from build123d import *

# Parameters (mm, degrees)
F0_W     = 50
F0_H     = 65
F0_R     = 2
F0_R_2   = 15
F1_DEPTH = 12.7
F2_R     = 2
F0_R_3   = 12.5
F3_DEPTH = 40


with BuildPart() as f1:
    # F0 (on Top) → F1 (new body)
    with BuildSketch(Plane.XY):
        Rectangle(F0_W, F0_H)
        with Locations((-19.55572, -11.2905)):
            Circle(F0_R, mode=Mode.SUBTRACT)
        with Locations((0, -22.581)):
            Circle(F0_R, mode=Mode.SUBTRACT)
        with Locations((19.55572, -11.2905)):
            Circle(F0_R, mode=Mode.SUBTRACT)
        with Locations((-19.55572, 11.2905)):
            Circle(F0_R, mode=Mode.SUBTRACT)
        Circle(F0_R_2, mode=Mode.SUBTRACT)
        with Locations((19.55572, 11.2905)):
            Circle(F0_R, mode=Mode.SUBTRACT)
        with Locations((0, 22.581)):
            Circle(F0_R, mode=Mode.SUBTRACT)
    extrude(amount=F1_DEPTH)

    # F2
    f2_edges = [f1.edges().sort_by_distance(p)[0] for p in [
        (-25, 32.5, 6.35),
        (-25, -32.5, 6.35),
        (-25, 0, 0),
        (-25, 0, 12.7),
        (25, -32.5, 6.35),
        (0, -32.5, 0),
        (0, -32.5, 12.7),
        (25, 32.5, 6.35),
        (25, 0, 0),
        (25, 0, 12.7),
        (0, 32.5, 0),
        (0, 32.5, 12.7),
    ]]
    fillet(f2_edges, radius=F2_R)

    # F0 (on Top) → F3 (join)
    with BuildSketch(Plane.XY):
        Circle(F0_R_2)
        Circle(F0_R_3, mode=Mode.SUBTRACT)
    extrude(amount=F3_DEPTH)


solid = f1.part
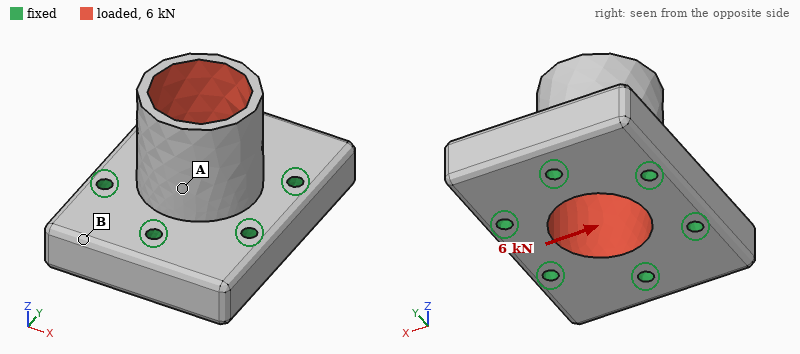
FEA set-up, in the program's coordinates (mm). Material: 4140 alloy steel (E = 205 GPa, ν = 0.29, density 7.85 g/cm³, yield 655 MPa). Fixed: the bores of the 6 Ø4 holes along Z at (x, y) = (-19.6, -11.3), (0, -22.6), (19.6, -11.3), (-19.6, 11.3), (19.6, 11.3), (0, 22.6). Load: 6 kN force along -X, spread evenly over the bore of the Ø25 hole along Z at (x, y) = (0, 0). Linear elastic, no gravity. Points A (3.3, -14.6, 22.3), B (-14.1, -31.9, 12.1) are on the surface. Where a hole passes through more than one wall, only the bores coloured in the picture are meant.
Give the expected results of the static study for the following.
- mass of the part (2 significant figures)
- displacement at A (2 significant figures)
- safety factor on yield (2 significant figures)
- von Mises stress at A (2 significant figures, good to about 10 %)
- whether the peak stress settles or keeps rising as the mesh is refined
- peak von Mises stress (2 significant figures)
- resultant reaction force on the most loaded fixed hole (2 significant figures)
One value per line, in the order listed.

310 g
5.6 µm
11
37 MPa
settles
60 MPa
1.6 kN
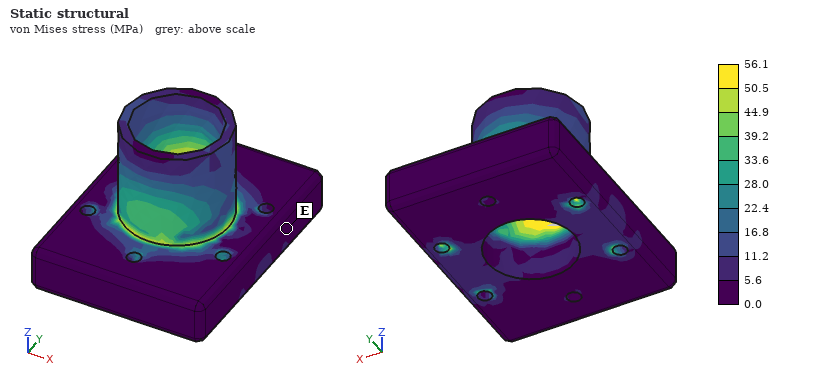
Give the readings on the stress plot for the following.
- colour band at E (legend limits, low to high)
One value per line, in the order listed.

0.0 to 5.6 MPa
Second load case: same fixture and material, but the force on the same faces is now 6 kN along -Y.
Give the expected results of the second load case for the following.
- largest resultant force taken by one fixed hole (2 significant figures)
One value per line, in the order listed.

1.8 kN
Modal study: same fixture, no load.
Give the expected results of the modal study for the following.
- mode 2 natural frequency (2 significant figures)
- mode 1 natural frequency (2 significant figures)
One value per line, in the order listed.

13 kHz
13 kHz
